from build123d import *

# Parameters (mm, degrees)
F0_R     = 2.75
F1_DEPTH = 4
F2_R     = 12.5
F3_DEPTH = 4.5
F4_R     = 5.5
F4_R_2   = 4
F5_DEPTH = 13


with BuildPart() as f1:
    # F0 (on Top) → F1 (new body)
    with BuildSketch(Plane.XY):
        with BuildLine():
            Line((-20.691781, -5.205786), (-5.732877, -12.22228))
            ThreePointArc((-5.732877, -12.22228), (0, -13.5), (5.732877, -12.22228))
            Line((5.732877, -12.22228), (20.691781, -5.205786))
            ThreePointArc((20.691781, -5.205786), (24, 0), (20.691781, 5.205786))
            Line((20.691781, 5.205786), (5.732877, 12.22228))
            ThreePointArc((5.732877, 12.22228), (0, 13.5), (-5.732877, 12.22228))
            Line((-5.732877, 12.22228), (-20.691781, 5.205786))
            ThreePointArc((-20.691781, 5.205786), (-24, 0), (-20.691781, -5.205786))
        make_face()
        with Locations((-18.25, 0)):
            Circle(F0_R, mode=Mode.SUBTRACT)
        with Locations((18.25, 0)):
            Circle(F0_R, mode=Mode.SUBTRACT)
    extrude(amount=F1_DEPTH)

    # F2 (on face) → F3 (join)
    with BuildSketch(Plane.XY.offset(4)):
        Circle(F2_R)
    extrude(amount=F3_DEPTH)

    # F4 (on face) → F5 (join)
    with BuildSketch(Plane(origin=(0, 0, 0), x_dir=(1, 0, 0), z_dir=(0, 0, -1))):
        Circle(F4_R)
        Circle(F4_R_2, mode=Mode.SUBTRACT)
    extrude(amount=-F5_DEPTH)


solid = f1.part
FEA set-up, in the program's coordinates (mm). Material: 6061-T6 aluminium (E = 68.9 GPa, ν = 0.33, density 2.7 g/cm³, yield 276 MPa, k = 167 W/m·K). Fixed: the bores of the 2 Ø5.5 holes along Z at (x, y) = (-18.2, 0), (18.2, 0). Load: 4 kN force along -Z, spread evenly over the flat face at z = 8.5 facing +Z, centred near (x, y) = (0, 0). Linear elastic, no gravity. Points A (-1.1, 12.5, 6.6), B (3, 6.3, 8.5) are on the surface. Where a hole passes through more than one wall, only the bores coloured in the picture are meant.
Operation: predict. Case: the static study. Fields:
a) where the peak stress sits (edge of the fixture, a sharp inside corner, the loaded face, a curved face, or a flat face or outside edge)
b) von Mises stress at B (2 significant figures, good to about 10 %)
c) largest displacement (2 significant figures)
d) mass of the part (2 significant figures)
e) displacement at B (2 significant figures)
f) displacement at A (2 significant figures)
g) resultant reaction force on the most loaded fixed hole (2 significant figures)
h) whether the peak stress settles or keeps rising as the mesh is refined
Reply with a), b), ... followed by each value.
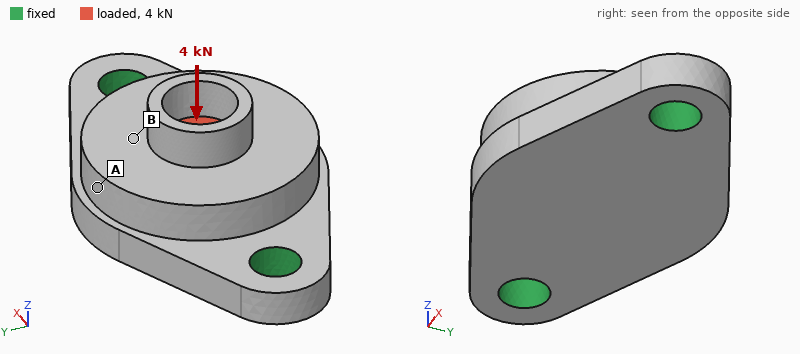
a) edge of the fixture
b) 59 MPa
c) 40 µm
d) 15 g
e) 34 µm
f) 37 µm
g) 2.5 kN
h) keeps rising
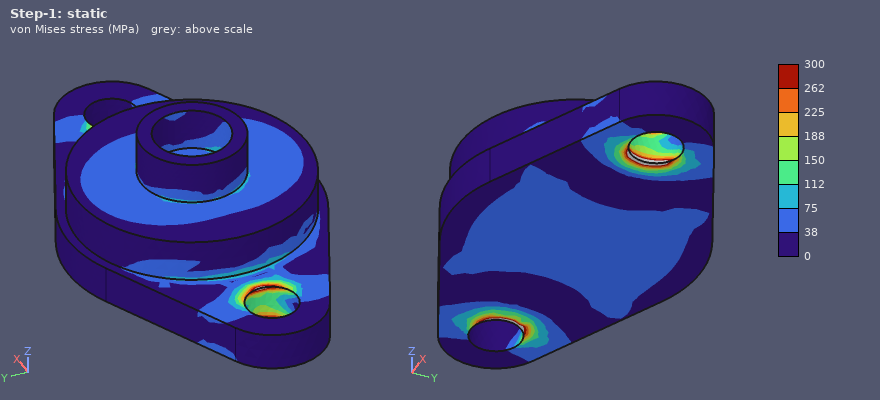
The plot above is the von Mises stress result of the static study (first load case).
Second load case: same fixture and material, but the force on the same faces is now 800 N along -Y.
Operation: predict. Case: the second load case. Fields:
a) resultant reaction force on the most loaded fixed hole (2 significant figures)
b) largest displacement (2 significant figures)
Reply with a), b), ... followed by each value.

a) 400 N
b) 25 µm
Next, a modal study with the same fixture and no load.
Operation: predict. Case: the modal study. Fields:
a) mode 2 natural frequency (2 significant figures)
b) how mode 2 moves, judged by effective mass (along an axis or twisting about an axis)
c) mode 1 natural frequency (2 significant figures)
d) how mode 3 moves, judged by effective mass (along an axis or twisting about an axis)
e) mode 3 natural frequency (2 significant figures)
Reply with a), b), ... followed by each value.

a) 16 kHz
b) along Z
c) 11 kHz
d) along Y
e) 26 kHz
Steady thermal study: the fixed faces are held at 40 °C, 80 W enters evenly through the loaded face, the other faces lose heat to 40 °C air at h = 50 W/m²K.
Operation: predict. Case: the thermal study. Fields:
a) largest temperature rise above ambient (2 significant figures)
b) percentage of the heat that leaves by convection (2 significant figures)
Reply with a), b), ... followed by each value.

a) 62 K
b) 4.3 %
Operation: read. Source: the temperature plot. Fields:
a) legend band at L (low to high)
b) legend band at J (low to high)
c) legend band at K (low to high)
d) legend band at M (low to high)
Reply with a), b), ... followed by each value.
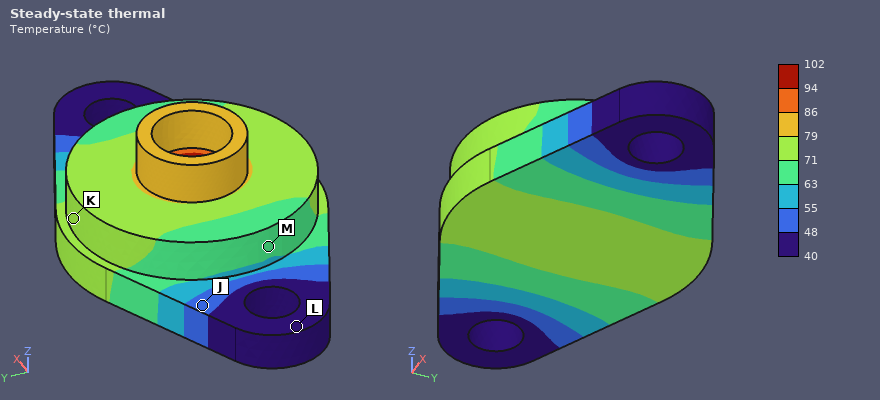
a) 40 to 48 °C
b) 48 to 55 °C
c) 71 to 79 °C
d) 63 to 71 °C
